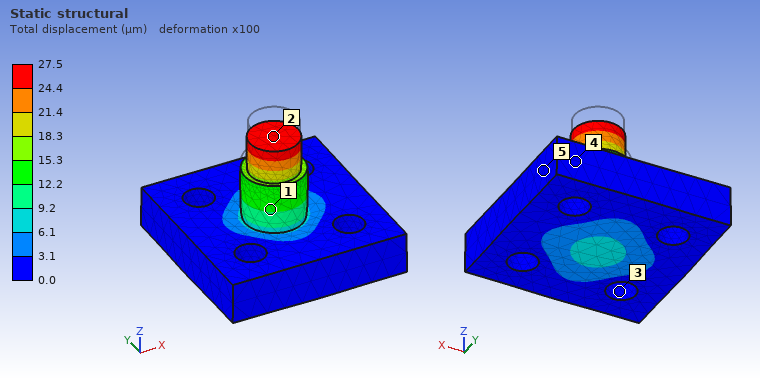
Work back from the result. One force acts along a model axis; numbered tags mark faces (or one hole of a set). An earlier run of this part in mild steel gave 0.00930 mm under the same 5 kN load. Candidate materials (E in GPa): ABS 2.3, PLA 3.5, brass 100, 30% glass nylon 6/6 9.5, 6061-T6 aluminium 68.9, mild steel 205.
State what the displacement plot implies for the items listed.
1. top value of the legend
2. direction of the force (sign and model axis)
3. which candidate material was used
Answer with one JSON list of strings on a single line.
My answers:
["27.5 µm", "-Z", "6061-T6 aluminium"]
